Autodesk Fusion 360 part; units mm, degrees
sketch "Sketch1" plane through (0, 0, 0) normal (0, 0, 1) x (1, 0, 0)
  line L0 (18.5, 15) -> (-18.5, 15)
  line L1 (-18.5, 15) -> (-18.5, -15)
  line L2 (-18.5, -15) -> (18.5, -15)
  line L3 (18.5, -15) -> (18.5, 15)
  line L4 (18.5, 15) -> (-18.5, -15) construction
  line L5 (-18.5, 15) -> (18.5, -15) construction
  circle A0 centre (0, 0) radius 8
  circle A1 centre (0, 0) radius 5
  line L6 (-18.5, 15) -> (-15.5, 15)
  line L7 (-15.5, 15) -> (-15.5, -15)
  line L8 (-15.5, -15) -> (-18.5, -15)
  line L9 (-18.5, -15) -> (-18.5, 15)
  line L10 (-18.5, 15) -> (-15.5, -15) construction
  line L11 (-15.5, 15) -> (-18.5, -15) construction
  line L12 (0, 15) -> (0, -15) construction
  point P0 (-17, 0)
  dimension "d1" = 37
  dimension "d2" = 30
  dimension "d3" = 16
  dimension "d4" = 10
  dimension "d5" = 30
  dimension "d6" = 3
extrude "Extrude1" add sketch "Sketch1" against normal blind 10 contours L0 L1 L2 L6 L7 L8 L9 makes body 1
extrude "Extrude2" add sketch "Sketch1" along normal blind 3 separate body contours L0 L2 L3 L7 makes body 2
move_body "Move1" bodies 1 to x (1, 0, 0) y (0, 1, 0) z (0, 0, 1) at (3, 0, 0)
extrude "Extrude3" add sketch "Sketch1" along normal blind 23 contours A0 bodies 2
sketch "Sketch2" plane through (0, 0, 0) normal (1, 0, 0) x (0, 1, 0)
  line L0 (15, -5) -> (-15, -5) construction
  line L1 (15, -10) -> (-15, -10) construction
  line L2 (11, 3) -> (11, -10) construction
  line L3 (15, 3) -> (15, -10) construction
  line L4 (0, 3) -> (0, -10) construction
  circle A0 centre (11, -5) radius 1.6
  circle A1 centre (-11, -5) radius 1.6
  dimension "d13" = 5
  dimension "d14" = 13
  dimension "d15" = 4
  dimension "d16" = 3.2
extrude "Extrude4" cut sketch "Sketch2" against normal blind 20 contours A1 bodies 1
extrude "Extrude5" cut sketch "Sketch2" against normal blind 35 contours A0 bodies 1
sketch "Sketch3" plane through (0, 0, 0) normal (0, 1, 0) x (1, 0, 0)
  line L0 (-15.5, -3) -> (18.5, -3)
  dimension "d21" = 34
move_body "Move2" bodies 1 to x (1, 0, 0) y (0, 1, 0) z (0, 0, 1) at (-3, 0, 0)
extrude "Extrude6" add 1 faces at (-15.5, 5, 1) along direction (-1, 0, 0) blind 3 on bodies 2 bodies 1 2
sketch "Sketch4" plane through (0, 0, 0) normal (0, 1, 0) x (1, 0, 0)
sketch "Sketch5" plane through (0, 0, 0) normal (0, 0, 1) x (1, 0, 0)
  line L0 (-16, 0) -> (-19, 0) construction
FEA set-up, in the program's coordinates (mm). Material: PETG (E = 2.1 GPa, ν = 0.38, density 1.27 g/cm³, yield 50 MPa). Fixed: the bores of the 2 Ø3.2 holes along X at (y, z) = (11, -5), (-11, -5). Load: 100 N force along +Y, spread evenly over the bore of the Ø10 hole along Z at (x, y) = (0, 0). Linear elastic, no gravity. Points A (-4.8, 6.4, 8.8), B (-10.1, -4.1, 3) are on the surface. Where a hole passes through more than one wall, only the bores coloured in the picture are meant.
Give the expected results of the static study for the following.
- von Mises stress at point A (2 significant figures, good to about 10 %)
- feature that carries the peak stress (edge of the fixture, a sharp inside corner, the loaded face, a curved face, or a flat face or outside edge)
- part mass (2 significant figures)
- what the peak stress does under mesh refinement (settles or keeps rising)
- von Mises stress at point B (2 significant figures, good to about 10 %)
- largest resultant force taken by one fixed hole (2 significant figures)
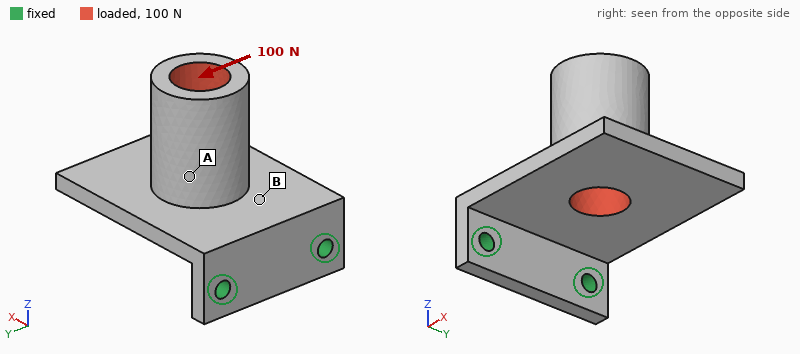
2.6 MPa
edge of the fixture
8.1 g
keeps rising
11 MPa
110 N
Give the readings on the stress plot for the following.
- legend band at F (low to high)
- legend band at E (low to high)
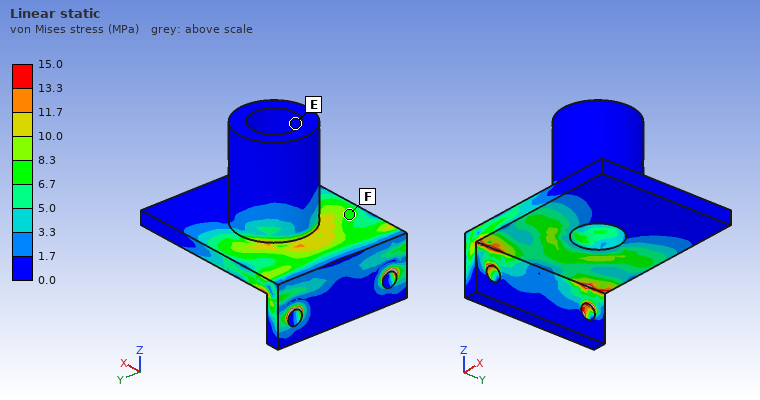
6.7 to 8.3 MPa
0.0 to 1.7 MPa
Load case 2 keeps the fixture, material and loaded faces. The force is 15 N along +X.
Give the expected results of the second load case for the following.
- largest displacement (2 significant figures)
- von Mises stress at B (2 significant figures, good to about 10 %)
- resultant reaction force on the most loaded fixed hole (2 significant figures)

0.66 mm
3.3 MPa
7.5 N
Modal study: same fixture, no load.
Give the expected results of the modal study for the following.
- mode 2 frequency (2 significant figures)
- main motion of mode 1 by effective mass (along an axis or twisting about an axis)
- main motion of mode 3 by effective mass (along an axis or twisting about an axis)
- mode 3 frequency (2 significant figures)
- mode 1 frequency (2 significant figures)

1000 Hz
along Z
along Y
1400 Hz
300 Hz
